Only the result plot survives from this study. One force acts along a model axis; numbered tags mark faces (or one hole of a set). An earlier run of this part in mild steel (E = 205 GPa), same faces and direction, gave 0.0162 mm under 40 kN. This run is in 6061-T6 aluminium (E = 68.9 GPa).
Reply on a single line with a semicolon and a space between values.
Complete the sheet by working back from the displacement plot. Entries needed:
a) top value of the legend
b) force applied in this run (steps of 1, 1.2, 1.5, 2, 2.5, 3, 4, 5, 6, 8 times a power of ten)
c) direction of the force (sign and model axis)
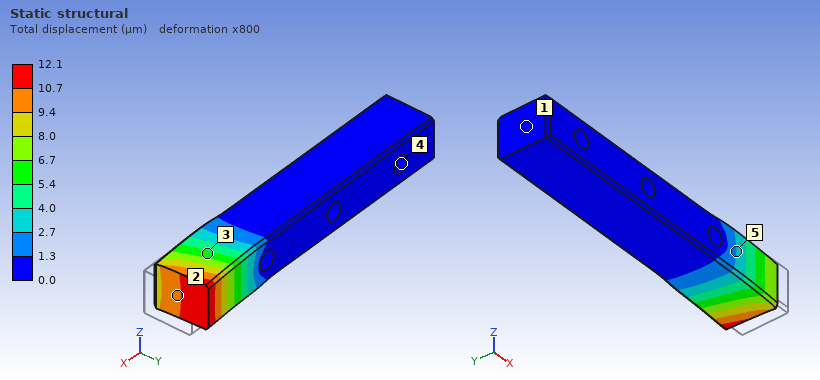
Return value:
12.1 µm; 10 kN; -X
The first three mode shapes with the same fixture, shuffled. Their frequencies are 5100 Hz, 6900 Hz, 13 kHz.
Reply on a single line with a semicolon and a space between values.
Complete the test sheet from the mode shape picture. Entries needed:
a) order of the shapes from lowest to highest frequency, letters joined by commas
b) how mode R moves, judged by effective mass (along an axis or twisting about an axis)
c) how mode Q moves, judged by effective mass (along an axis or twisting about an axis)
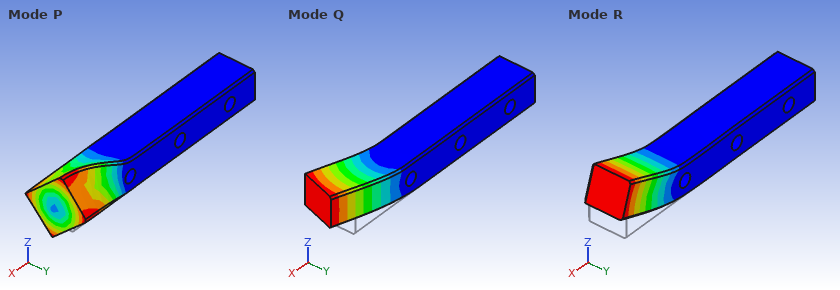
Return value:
R, Q, P; along Z; along Y
